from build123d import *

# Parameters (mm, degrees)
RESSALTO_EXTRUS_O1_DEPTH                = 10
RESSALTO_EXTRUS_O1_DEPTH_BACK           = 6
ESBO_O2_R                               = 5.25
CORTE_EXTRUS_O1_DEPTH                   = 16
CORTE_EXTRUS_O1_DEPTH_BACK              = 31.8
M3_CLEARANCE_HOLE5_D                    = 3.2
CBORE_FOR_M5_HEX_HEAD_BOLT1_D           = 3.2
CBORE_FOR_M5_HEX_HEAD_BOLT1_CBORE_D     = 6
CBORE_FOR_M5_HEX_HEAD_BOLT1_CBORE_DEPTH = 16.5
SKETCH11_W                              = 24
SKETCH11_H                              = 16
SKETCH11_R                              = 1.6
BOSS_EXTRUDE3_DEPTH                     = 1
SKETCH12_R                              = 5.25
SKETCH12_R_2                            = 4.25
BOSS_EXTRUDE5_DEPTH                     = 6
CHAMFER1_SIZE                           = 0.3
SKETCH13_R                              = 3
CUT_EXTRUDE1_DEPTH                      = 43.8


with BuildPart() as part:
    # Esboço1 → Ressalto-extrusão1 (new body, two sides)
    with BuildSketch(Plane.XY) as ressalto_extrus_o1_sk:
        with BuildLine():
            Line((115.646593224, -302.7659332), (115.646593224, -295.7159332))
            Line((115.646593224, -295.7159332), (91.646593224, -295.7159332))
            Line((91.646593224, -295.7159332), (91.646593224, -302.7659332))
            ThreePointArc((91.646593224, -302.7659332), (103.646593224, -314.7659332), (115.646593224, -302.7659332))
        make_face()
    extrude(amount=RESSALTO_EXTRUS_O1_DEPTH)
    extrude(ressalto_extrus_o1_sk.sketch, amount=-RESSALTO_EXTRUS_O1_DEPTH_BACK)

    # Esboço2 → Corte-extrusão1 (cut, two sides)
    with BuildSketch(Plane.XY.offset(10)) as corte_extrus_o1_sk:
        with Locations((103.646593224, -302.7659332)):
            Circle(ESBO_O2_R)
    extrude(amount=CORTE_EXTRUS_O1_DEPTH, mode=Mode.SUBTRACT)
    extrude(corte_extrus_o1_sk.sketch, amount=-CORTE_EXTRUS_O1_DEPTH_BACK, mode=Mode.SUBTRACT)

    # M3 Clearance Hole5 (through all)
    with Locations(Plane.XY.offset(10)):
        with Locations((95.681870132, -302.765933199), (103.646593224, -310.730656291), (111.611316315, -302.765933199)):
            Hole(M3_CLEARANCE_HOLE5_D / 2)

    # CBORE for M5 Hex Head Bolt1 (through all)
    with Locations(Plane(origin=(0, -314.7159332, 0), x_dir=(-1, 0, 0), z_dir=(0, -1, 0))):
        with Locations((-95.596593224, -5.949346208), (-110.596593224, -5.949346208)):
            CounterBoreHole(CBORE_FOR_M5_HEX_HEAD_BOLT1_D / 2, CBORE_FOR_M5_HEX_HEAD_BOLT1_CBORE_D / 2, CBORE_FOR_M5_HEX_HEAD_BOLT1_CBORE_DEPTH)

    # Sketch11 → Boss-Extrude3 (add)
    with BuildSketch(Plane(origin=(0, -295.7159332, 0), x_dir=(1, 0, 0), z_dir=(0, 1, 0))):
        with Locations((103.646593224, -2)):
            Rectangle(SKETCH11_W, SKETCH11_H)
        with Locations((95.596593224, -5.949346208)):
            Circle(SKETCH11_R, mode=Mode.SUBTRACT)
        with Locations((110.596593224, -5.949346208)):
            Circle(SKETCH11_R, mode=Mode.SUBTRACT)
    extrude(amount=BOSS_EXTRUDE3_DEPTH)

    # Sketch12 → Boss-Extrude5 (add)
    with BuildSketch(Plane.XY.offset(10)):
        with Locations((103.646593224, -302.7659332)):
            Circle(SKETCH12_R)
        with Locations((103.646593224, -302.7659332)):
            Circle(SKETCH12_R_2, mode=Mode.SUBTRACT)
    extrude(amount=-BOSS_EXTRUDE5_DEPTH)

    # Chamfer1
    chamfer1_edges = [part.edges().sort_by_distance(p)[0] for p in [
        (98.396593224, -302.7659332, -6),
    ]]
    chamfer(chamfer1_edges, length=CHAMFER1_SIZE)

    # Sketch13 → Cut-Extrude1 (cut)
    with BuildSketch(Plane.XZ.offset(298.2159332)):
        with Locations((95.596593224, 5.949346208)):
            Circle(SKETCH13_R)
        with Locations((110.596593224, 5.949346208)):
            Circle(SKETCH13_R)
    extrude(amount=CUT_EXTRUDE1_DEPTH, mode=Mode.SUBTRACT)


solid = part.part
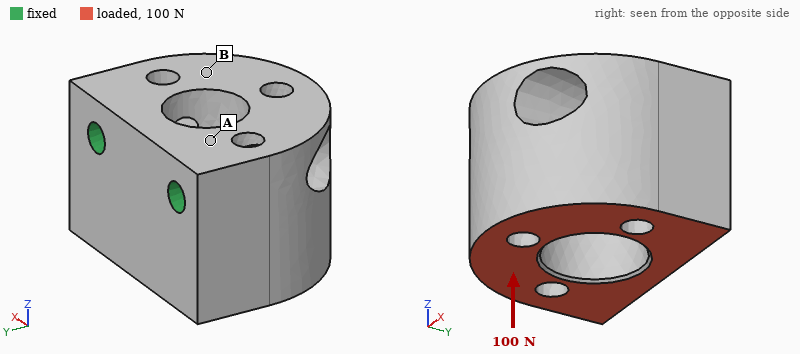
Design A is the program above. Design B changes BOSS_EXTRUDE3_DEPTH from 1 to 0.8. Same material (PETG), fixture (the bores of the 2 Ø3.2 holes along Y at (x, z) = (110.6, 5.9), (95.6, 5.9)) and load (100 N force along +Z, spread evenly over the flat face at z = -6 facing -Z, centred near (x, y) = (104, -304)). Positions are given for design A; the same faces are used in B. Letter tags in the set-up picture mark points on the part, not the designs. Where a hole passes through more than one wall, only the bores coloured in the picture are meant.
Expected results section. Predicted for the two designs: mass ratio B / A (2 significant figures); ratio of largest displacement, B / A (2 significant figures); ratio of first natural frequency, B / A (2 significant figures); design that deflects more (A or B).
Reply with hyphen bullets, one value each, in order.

- 0.98
- 1.1
- 0.96
- B
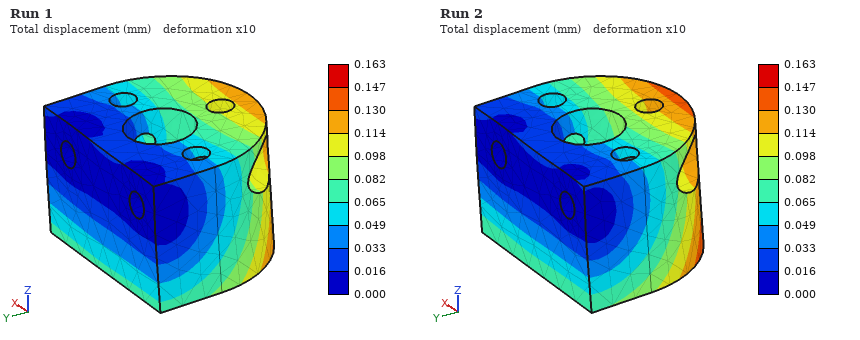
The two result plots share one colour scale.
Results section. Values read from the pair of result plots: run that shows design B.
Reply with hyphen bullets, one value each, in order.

- Run 2
